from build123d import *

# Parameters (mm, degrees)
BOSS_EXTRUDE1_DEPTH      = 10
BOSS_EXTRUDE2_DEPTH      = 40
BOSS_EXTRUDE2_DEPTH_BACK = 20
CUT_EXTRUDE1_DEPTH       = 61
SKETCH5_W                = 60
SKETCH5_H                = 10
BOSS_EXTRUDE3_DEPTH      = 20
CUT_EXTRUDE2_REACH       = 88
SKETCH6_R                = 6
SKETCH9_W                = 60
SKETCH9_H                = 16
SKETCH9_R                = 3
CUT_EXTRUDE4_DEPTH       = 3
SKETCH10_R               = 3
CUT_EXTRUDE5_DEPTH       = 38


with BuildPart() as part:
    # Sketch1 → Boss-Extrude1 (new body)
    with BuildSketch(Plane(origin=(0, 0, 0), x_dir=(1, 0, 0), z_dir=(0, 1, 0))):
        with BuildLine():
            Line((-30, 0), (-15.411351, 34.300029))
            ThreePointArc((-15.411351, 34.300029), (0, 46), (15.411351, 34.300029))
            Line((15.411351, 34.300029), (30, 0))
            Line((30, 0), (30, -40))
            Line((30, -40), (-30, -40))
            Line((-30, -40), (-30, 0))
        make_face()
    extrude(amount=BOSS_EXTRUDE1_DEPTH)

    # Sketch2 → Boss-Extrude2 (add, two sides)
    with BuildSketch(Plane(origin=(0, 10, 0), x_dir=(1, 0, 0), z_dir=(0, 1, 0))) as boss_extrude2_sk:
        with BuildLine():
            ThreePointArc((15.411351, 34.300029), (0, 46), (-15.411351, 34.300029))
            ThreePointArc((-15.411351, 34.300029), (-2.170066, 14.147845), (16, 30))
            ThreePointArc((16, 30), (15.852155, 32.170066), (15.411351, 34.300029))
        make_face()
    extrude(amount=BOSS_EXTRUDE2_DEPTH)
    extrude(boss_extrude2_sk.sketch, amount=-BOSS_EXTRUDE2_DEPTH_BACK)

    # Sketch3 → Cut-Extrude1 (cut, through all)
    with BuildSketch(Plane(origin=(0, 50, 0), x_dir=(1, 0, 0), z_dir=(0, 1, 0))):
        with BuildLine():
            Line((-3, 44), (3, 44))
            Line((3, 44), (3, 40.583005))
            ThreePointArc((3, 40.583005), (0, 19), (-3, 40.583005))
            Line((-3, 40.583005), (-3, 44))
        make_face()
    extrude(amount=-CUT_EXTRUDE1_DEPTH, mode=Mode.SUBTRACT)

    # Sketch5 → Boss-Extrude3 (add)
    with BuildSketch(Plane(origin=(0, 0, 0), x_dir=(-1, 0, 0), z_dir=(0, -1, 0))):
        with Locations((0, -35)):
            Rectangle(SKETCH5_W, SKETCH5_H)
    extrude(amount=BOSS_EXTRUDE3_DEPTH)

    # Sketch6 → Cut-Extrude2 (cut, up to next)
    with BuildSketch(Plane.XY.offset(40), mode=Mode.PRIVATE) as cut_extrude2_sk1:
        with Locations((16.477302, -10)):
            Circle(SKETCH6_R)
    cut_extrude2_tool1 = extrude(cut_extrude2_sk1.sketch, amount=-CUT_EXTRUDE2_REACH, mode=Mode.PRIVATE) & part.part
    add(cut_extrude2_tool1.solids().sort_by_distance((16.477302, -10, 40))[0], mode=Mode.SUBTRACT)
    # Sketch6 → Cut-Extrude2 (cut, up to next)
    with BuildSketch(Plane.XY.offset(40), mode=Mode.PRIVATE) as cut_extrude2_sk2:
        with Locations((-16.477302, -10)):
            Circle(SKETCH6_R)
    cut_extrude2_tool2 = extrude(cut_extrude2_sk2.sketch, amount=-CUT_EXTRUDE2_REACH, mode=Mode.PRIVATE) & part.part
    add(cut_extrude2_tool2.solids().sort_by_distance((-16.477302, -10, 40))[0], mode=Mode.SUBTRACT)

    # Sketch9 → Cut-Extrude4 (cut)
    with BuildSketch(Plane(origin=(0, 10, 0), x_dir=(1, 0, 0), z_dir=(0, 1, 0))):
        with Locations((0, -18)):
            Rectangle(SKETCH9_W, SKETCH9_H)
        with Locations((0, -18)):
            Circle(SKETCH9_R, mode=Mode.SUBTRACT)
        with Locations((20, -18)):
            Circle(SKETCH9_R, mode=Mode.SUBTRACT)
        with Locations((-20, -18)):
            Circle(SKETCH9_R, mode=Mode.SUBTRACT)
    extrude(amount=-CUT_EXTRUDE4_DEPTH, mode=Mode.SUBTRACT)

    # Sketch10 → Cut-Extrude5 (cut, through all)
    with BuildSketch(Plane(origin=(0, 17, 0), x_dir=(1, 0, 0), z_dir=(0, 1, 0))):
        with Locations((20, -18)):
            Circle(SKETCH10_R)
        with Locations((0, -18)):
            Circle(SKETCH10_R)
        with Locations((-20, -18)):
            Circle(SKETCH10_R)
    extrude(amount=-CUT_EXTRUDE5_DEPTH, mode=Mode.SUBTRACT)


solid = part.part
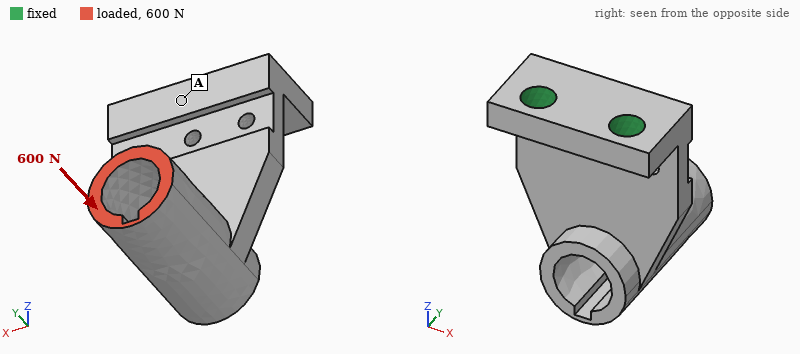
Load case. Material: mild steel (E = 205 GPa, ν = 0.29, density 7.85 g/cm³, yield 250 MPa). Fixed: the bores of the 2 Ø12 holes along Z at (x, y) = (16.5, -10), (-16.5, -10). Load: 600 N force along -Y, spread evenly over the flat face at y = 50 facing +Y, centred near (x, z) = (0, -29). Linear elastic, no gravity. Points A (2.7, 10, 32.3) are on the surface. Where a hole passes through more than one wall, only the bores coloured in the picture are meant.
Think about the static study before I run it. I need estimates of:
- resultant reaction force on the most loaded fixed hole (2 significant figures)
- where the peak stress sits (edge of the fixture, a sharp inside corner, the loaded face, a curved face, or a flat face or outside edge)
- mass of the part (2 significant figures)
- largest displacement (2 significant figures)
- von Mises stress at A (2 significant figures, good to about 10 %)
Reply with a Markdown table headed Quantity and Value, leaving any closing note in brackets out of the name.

| Quantity | Value |
|---|---|
| resultant reaction force on the most loaded fixed hole | 330 N |
| where the peak stress sits | a curved face |
| mass of the part | 510 g |
| largest displacement | 0.23 mm |
| von Mises stress at A | 17 MPa |
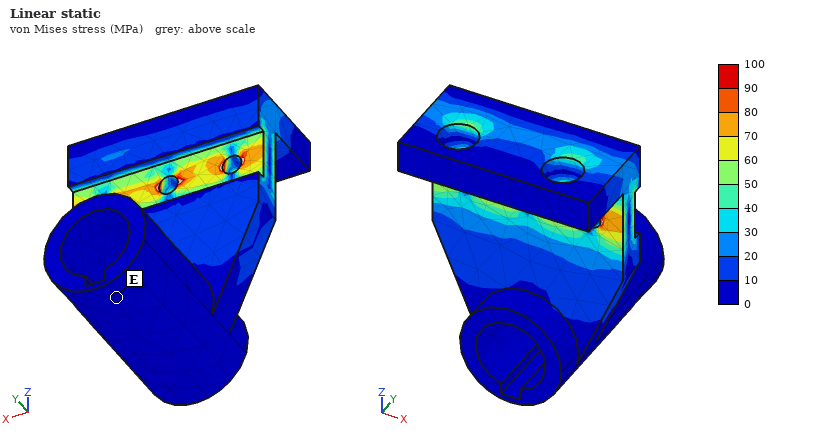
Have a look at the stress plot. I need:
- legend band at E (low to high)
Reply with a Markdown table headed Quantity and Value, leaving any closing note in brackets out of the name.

| Quantity | Value |
|---|---|
| legend band at E | 0 to 10 MPa |
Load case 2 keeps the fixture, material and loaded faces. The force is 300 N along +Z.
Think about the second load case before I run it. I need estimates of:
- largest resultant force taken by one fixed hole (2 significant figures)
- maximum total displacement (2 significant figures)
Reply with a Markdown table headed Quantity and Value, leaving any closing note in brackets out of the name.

| Quantity | Value |
|---|---|
| largest resultant force taken by one fixed hole | 150 N |
| maximum total displacement | 0.12 mm |
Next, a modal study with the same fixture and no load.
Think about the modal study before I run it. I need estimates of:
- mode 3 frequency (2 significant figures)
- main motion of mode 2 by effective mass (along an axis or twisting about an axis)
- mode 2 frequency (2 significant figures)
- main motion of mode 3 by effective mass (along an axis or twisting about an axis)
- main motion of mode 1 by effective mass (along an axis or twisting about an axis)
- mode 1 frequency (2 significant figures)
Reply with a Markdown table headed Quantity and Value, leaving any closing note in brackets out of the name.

| Quantity | Value |
|---|---|
| mode 3 frequency | 3400 Hz |
| main motion of mode 2 by effective mass | along X |
| mode 2 frequency | 2000 Hz |
| main motion of mode 3 by effective mass | along X |
| main motion of mode 1 by effective mass | along Y |
| mode 1 frequency | 630 Hz |
